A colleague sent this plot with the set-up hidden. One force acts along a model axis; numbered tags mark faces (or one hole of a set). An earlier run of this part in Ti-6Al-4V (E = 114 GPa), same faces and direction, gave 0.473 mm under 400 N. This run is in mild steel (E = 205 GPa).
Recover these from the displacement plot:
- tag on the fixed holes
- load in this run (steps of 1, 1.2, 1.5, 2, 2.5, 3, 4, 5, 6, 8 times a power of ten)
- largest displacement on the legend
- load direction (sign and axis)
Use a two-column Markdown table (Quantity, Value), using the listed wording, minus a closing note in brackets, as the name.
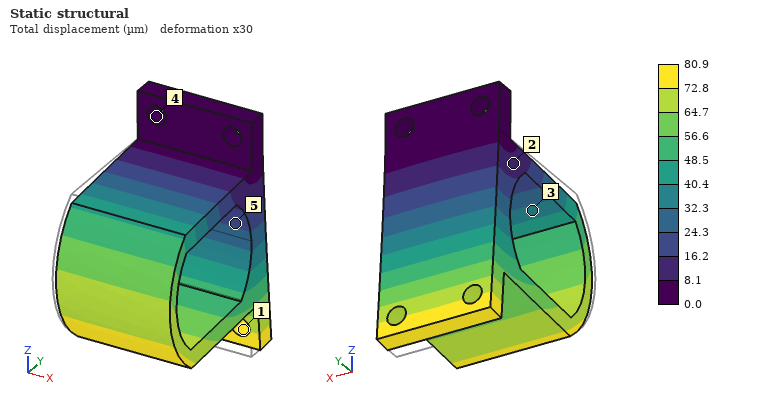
| Quantity | Value |
|---|---|
| tag on the fixed holes | 4 |
| load in this run | 120 N |
| largest displacement on the legend | 80.9 µm |
| load direction | +Y |
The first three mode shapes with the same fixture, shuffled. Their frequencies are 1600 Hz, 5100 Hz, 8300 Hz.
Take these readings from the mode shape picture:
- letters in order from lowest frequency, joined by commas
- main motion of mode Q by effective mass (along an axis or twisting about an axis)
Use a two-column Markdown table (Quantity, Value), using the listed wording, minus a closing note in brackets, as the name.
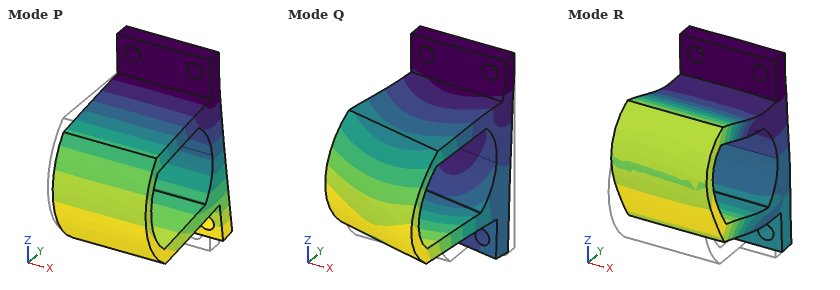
| Quantity | Value |
|---|---|
| letters in order from lowest frequency, joined by commas | P, Q, R |
| main motion of mode Q by effective mass | along X |
